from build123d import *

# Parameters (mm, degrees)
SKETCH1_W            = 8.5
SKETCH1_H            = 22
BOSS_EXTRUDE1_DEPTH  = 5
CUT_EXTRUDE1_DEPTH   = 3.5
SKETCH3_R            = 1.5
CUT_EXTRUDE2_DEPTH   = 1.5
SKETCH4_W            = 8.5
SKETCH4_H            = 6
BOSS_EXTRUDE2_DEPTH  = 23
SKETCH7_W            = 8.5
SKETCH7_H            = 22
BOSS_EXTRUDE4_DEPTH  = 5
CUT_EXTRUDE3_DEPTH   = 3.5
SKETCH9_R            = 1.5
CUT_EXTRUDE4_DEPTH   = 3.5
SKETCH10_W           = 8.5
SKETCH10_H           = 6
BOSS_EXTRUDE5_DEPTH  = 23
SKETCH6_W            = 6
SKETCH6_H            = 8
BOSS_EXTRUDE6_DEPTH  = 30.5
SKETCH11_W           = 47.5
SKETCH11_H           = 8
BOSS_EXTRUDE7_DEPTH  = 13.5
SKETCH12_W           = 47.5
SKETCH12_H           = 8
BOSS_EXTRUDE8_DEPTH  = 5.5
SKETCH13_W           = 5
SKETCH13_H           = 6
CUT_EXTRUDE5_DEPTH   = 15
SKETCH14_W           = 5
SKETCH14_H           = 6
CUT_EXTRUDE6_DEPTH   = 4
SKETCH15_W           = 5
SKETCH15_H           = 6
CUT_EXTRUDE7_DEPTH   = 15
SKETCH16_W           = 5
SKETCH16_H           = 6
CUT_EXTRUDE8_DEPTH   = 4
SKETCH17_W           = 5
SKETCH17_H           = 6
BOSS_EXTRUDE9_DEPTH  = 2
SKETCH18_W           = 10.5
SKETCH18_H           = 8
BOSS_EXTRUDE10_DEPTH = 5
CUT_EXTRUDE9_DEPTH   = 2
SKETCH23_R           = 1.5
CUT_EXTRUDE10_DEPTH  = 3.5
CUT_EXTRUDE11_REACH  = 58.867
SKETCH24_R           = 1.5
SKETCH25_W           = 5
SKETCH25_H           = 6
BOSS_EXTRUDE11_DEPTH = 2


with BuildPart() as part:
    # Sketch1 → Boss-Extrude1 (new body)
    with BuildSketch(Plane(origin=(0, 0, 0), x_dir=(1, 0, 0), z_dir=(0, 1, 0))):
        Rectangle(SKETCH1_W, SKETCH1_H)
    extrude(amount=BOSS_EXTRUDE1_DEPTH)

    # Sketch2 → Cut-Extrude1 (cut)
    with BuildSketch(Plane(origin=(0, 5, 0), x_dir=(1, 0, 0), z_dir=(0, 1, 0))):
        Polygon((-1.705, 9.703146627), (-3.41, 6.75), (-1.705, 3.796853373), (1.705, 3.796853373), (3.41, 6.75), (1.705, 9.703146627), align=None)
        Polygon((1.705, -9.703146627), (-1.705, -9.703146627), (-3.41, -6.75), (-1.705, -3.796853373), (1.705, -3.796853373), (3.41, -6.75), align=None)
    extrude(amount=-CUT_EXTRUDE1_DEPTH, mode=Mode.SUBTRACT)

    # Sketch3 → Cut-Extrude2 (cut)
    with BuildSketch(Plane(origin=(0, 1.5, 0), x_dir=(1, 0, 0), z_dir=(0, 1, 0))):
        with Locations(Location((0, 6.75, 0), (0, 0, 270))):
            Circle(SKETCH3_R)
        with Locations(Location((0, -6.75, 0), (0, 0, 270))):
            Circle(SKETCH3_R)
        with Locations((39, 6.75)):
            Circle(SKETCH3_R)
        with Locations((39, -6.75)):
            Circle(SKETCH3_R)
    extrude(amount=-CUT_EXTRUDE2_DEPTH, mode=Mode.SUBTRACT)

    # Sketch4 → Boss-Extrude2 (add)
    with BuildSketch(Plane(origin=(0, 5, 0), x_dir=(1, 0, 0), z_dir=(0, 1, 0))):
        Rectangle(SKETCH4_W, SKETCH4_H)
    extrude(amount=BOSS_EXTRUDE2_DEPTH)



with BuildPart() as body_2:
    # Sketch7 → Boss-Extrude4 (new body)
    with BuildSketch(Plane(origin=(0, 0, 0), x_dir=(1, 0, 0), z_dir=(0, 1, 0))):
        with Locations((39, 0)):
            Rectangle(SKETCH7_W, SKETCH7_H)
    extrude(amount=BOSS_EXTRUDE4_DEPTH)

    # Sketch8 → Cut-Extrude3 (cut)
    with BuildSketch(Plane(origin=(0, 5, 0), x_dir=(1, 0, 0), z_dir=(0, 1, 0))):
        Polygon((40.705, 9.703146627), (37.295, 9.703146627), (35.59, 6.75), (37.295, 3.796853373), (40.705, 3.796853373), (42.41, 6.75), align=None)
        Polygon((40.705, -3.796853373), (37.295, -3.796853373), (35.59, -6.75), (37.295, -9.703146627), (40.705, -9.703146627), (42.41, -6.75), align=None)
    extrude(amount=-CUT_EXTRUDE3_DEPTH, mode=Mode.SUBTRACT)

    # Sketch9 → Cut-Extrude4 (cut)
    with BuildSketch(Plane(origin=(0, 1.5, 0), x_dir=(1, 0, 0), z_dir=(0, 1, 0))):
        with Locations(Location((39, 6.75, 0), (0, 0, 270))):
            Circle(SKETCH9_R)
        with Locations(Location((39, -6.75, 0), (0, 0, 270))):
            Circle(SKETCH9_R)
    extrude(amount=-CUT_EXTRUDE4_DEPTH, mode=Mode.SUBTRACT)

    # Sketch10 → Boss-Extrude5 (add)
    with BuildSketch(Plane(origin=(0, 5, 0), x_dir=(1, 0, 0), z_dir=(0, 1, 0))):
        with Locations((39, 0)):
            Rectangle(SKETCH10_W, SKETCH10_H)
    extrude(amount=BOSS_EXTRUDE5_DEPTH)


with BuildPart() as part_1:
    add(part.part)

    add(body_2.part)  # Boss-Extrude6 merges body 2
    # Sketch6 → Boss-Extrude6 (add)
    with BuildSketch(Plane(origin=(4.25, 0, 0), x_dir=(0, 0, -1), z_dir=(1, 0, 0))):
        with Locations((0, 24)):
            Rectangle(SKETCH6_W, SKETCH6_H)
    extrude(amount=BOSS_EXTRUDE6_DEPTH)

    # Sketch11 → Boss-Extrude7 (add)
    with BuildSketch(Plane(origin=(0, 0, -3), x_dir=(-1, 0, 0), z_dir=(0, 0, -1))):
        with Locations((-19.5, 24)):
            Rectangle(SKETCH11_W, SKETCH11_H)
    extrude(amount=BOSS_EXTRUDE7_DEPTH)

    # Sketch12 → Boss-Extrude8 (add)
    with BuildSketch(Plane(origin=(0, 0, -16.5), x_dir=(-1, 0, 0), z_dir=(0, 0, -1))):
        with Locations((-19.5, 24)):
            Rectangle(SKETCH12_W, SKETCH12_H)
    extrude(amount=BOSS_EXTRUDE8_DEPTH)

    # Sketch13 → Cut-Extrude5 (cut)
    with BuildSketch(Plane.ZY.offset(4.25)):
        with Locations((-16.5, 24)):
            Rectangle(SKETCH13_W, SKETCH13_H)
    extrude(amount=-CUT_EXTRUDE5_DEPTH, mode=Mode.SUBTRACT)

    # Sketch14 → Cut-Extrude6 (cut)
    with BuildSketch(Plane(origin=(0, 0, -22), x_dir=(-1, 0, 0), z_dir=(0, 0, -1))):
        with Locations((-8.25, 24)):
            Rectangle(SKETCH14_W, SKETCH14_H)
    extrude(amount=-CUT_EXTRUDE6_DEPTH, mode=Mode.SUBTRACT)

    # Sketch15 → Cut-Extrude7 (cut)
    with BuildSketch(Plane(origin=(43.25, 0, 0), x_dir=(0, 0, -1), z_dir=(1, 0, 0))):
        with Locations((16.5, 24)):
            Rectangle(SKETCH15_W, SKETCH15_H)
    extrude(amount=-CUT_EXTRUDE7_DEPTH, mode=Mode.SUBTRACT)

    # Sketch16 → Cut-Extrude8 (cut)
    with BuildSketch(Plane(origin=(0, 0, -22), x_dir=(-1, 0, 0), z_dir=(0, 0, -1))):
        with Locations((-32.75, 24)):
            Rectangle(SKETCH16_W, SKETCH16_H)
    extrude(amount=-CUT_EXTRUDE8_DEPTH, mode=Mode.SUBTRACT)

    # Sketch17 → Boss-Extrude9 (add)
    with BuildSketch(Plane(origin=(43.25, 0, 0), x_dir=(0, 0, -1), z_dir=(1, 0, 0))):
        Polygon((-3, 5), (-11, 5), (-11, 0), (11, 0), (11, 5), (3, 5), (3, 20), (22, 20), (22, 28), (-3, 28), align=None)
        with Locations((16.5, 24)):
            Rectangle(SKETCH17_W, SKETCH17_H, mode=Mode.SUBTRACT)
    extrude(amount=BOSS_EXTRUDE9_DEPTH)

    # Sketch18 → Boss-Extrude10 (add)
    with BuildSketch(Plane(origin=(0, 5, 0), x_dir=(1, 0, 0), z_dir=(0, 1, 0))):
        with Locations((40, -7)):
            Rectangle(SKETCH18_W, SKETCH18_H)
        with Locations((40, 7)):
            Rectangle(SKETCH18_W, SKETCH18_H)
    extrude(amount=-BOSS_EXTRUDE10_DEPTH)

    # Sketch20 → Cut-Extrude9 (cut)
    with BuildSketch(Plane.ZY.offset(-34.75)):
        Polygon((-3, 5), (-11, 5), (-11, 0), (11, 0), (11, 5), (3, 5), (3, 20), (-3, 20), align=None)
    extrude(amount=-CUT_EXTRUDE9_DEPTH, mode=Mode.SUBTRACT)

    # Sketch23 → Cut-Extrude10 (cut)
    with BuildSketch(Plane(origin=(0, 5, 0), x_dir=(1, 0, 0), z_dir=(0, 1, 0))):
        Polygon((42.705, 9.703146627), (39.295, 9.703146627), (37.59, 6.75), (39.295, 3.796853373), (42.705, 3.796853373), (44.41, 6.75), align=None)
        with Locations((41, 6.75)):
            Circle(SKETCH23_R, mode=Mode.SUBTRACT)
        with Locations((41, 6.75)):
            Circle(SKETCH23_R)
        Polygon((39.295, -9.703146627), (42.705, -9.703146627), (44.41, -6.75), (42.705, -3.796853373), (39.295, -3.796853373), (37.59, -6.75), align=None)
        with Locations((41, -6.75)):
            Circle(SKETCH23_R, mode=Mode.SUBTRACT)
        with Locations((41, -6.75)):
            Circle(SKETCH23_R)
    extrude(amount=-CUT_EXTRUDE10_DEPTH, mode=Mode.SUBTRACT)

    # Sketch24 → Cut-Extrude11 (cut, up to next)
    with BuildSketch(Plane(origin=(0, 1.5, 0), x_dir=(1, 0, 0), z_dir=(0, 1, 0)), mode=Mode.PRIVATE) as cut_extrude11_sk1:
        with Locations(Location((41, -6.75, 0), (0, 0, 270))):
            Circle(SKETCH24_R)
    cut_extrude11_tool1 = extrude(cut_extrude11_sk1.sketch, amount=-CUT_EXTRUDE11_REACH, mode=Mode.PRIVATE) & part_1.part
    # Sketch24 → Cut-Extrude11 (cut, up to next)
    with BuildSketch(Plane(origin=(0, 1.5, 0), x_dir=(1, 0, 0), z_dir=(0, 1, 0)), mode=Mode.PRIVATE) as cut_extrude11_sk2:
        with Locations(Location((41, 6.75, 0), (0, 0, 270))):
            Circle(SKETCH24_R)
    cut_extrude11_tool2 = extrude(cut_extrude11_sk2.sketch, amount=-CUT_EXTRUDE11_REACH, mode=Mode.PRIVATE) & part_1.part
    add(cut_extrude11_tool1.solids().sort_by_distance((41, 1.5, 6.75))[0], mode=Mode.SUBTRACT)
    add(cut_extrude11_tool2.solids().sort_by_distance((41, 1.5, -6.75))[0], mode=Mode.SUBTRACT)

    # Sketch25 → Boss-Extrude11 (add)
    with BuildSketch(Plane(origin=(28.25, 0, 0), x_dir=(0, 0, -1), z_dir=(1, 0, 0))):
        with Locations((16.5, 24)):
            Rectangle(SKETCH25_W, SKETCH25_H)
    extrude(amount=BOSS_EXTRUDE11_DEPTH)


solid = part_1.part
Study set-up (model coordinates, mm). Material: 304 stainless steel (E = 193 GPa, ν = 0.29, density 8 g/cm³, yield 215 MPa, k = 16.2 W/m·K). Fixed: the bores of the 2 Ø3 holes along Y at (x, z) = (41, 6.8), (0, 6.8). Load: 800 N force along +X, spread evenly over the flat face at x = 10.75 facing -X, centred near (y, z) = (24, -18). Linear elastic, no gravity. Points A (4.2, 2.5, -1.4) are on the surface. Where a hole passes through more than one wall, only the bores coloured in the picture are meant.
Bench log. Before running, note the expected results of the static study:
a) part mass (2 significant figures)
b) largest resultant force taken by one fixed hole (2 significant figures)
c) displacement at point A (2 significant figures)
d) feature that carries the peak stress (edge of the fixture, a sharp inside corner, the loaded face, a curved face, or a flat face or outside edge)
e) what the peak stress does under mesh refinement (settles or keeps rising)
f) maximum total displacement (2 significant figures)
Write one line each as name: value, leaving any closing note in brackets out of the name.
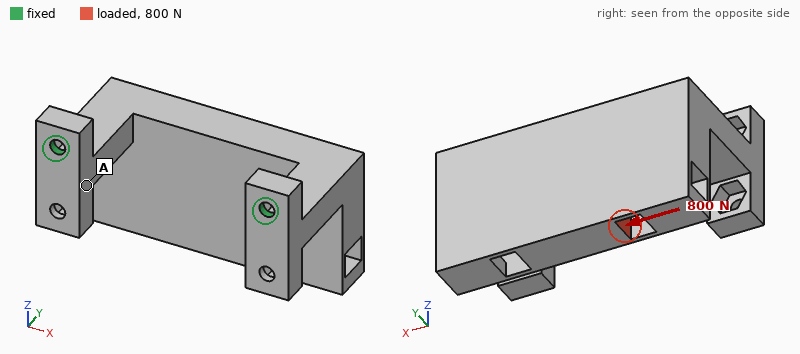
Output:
part mass: 94 g
largest resultant force taken by one fixed hole: 650 N
displacement at point A: 15 µm
feature that carries the peak stress: edge of the fixture
what the peak stress does under mesh refinement: keeps rising
maximum total displacement: 66 µm
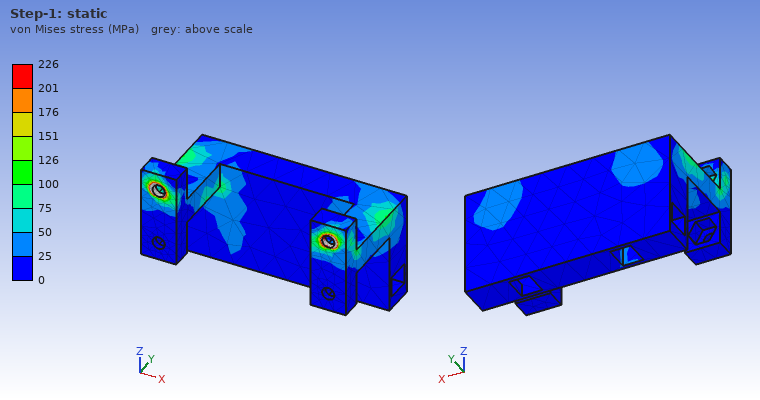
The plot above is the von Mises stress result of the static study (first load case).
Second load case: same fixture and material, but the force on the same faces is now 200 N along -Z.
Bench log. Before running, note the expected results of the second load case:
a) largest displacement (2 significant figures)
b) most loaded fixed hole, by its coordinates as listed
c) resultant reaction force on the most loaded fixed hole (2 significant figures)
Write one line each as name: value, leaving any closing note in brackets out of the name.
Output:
largest displacement: 0.14 mm
most loaded fixed hole, by its coordinates as listed: (0, 6.8)
resultant reaction force on the most loaded fixed hole: 140 N
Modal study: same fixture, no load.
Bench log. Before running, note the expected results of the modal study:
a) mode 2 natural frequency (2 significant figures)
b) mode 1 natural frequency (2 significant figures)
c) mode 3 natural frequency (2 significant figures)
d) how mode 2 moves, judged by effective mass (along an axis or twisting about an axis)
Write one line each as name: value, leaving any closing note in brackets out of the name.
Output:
mode 2 natural frequency: 2600 Hz
mode 1 natural frequency: 760 Hz
mode 3 natural frequency: 3100 Hz
how mode 2 moves, judged by effective mass: along X
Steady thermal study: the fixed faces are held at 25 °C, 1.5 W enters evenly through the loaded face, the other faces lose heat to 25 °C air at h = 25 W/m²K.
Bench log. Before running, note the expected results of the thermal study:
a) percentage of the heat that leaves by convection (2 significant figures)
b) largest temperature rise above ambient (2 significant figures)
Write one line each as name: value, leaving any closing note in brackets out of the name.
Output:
percentage of the heat that leaves by convection: 77 %
largest temperature rise above ambient: 20 K
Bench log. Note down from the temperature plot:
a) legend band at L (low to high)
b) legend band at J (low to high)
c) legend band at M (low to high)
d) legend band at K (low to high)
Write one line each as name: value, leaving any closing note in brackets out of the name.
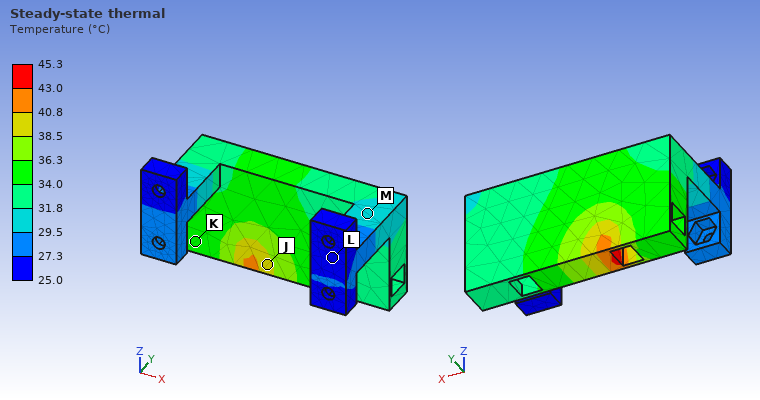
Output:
legend band at L: 25.0 to 27.3 °C
legend band at J: 38.5 to 40.8 °C
legend band at M: 29.5 to 31.8 °C
legend band at K: 34.0 to 36.3 °C
